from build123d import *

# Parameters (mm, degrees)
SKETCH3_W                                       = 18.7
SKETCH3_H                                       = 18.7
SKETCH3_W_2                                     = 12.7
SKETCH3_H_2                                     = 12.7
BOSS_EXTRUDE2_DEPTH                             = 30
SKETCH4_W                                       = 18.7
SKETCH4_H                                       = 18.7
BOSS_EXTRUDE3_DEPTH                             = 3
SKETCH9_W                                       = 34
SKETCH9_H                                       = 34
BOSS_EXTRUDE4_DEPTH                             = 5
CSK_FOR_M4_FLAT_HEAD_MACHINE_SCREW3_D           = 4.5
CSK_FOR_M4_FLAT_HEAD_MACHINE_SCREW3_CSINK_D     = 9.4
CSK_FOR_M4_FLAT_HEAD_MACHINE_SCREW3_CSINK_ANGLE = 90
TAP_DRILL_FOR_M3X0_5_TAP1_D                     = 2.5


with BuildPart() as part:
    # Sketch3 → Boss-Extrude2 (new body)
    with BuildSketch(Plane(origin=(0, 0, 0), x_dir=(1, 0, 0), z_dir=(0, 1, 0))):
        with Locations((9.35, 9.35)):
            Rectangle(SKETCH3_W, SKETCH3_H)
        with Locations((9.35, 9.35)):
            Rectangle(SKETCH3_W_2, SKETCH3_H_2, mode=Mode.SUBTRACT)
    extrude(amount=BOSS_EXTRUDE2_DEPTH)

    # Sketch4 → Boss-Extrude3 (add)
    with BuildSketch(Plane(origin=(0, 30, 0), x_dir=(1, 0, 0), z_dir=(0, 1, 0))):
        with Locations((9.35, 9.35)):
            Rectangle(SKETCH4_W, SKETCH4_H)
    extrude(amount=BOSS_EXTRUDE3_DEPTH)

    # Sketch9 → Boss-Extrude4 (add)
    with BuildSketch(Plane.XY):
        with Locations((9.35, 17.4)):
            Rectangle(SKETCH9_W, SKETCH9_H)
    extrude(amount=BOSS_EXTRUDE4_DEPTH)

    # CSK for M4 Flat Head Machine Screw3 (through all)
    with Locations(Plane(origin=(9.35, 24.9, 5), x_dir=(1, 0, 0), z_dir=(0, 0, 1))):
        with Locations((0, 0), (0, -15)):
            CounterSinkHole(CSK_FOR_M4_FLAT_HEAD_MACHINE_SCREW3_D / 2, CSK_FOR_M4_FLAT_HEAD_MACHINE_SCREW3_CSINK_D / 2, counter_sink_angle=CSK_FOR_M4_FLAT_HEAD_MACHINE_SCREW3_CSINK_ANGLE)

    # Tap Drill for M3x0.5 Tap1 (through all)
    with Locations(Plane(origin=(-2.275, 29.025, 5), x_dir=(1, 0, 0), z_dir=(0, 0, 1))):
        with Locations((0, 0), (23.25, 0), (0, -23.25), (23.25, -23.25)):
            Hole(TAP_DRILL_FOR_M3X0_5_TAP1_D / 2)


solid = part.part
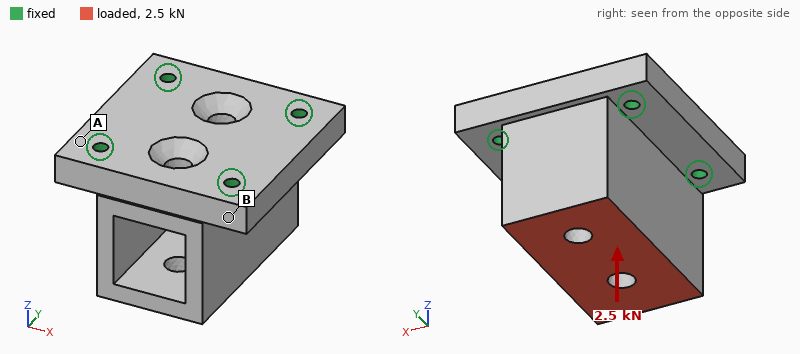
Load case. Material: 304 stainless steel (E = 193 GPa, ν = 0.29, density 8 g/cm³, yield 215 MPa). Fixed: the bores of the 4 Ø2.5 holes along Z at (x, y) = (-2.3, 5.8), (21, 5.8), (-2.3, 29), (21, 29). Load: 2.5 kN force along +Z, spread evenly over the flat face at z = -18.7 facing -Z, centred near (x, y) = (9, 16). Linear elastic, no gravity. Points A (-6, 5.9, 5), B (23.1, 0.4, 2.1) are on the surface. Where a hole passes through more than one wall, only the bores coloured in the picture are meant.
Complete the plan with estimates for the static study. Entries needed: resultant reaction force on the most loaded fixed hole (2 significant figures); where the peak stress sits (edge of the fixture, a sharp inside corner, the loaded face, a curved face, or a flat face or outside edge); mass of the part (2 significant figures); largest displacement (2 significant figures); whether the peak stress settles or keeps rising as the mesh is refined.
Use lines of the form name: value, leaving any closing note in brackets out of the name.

resultant reaction force on the most loaded fixed hole: 690 N
where the peak stress sits: edge of the fixture
mass of the part: 95 g
largest displacement: 5.9 µm
whether the peak stress settles or keeps rising as the mesh is refined: keeps rising
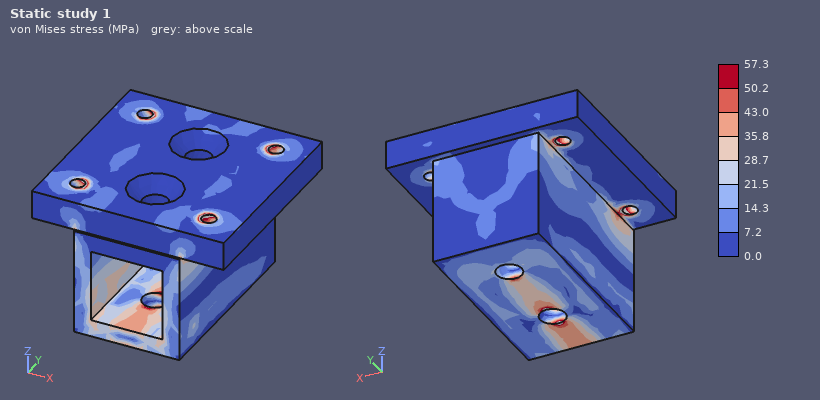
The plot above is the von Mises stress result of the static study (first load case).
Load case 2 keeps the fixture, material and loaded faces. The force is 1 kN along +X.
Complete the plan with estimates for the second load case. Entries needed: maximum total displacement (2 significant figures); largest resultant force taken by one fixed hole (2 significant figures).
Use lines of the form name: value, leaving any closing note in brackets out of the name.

maximum total displacement: 14 µm
largest resultant force taken by one fixed hole: 780 N
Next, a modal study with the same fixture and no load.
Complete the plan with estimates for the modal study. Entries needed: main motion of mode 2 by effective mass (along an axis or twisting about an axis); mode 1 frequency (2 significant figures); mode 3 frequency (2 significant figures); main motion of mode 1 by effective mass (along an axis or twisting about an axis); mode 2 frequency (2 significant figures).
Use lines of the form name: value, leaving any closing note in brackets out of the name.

main motion of mode 2 by effective mass: along Y
mode 1 frequency: 11 kHz
mode 3 frequency: 24 kHz
main motion of mode 1 by effective mass: along X
mode 2 frequency: 17 kHz
